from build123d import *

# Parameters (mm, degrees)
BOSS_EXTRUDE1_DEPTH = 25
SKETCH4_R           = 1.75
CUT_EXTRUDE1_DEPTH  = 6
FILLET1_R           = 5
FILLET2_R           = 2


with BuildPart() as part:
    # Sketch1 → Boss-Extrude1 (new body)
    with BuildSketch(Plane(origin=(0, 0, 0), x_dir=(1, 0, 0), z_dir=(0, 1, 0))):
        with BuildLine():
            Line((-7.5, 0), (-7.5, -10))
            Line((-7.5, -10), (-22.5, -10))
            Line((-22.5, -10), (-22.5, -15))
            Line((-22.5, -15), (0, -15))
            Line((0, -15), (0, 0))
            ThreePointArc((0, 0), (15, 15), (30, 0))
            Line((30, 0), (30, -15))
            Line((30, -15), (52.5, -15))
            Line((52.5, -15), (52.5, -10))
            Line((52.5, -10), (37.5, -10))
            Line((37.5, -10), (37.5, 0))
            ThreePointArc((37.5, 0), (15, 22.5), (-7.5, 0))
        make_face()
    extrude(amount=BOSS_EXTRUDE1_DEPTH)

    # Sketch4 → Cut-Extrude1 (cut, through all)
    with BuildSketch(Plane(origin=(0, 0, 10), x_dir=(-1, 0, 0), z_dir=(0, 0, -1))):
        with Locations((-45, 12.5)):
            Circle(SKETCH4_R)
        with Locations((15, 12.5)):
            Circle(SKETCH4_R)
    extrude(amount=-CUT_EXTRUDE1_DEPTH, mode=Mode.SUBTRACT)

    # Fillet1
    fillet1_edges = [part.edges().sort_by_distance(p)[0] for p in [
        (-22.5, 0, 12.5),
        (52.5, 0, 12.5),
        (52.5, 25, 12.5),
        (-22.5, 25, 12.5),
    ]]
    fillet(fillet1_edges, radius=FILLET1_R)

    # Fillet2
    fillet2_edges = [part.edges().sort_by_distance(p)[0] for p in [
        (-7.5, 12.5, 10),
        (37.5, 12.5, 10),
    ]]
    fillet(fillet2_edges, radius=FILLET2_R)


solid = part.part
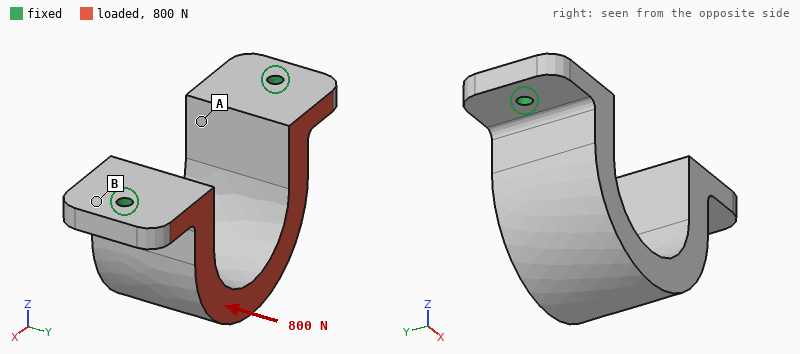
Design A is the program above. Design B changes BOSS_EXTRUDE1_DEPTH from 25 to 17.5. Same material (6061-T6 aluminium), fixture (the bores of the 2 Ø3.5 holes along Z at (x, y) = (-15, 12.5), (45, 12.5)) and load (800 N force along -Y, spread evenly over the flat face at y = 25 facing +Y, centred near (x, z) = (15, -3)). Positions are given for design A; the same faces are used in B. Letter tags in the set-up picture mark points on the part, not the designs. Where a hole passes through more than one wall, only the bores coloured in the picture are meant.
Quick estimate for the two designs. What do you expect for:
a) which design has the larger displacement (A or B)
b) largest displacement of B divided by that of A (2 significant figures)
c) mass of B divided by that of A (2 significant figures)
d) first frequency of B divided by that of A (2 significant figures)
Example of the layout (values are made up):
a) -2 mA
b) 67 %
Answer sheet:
a) B
b) 1.4
c) 0.70
d) 1.0
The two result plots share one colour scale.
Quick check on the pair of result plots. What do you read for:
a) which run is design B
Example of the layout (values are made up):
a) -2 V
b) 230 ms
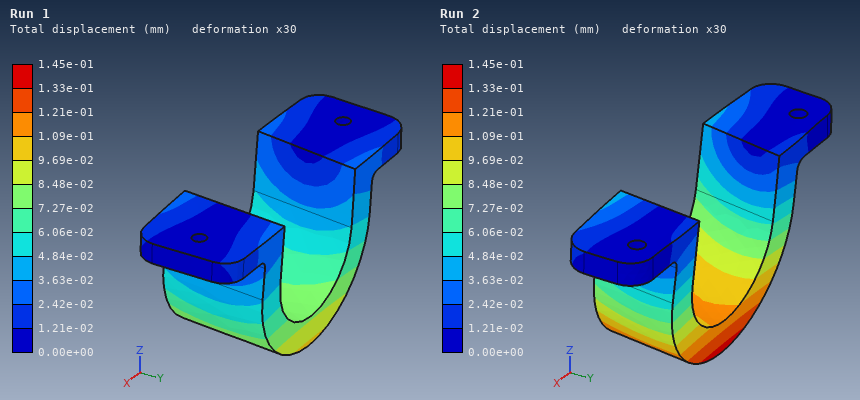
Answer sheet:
a) Run 2
